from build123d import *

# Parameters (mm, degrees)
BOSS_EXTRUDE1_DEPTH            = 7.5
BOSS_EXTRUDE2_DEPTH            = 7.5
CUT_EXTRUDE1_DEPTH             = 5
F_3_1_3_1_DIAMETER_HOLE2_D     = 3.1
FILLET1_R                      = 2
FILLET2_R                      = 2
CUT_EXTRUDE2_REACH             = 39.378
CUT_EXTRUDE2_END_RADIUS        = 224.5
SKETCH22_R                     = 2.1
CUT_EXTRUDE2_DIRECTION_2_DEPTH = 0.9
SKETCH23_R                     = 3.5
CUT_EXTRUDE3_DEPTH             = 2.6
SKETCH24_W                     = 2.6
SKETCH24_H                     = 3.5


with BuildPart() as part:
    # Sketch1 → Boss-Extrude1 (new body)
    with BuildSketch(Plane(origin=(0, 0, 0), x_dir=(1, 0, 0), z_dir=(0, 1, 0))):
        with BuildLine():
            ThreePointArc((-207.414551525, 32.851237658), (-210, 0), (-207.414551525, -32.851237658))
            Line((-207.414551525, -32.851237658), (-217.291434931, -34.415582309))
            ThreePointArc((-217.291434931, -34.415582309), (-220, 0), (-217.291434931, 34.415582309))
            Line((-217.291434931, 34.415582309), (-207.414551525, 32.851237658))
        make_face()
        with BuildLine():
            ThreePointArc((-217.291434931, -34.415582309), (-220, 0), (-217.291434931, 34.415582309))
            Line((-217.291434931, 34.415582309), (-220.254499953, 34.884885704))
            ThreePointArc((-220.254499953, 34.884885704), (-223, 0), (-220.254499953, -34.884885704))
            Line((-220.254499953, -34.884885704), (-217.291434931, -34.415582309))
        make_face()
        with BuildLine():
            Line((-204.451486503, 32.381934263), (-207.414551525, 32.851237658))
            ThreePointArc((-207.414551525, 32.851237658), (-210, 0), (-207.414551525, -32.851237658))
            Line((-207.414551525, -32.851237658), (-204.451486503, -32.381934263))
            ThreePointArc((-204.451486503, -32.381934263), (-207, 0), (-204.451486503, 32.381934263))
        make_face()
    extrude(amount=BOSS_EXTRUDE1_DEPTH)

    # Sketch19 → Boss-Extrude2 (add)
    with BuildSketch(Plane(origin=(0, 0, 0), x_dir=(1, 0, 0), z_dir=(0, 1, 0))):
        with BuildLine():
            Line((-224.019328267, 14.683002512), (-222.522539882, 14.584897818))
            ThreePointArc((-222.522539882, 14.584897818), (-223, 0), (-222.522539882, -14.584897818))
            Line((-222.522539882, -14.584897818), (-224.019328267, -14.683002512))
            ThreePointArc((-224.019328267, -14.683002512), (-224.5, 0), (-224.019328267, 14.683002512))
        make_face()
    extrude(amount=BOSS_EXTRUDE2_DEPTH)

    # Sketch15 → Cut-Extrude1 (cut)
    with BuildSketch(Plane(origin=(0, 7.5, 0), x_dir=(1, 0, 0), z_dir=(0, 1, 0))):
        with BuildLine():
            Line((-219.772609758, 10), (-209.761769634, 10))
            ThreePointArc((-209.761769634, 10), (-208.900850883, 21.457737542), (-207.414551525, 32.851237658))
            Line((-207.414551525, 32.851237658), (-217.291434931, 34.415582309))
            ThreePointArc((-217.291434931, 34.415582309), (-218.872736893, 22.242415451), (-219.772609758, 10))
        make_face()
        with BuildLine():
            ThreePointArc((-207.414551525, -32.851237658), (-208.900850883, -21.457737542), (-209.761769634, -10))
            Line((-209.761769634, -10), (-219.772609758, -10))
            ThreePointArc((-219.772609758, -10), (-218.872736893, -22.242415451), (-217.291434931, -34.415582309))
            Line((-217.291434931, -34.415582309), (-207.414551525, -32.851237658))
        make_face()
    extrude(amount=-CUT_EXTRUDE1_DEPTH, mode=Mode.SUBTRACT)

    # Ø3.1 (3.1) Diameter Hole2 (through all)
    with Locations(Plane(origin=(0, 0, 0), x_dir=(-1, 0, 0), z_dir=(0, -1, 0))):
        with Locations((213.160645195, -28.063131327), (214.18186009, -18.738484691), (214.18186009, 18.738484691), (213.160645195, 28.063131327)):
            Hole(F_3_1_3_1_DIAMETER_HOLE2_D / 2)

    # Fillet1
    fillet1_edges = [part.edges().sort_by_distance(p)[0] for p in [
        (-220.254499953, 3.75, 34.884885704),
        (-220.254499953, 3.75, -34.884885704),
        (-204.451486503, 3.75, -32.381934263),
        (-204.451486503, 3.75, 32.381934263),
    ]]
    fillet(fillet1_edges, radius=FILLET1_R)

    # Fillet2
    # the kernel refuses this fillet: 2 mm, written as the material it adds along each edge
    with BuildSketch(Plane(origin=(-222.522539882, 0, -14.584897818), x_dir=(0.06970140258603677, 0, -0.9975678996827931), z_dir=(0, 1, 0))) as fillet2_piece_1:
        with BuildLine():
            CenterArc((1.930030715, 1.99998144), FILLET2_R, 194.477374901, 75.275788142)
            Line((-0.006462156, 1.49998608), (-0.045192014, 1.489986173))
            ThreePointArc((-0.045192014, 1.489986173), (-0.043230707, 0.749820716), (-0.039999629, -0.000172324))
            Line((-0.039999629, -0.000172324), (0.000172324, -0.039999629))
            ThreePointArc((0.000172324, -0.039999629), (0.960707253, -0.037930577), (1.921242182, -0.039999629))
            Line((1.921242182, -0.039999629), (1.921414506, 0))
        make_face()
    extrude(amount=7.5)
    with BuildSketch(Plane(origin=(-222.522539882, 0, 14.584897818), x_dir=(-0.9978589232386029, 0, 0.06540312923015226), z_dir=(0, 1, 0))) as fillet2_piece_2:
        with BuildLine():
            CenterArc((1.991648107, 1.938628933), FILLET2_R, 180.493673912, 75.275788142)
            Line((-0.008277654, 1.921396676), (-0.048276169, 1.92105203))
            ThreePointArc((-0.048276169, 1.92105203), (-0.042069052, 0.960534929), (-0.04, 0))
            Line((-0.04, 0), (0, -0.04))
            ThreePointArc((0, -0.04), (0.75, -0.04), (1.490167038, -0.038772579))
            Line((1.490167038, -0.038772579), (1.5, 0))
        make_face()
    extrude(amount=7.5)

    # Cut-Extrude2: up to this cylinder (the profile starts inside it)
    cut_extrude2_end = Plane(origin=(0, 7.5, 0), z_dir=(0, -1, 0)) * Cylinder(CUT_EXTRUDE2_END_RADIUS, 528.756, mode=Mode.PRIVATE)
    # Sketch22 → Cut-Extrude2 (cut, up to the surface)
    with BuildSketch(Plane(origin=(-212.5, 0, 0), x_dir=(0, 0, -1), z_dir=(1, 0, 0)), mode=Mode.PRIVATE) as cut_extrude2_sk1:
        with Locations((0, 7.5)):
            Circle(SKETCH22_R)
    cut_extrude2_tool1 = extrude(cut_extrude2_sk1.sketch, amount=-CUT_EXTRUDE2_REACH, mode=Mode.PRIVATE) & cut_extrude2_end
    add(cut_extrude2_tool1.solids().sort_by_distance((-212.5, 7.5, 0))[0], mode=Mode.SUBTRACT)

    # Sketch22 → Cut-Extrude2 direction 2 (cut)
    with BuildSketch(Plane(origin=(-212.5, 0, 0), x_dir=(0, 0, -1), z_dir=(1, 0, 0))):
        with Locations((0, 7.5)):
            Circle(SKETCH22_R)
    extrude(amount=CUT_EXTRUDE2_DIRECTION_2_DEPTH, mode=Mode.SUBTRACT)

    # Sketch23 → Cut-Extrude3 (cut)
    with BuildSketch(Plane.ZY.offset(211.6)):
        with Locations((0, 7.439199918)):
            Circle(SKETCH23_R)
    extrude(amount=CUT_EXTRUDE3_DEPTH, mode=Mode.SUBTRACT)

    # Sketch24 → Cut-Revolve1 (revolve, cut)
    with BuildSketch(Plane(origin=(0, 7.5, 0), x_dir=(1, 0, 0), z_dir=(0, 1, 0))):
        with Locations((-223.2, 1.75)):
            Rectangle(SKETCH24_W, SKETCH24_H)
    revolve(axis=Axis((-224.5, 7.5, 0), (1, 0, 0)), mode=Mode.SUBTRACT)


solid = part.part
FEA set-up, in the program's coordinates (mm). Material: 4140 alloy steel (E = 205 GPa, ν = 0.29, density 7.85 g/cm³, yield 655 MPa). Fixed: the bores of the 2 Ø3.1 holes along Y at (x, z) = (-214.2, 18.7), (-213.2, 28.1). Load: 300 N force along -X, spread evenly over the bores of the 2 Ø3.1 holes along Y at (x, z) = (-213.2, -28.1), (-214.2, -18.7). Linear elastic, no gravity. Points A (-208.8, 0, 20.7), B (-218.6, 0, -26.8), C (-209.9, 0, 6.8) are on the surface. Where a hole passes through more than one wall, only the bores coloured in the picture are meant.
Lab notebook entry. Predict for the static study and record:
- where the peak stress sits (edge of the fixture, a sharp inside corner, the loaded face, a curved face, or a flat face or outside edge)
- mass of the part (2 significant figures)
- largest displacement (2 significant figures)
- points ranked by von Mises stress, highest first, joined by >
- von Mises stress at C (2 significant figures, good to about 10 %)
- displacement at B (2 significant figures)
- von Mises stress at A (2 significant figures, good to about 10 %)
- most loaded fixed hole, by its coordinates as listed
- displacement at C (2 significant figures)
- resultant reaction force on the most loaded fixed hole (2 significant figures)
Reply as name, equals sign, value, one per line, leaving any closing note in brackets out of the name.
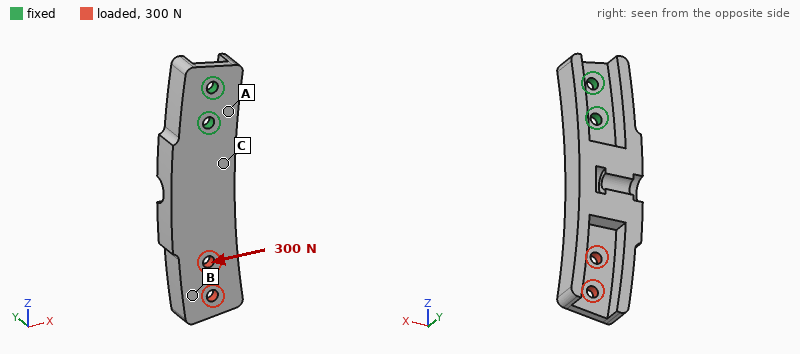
where the peak stress sits = edge of the fixture
mass of the part = 46 g
largest displacement = 52 µm
points ranked by von Mises stress, highest first, joined by > = A > C > B
von Mises stress at C = 24 MPa
displacement at B = 44 µm
von Mises stress at A = 40 MPa
most loaded fixed hole, by its coordinates as listed = (-214.2, 18.7)
displacement at C = 9.7 µm
resultant reaction force on the most loaded fixed hole = 1.2 kN
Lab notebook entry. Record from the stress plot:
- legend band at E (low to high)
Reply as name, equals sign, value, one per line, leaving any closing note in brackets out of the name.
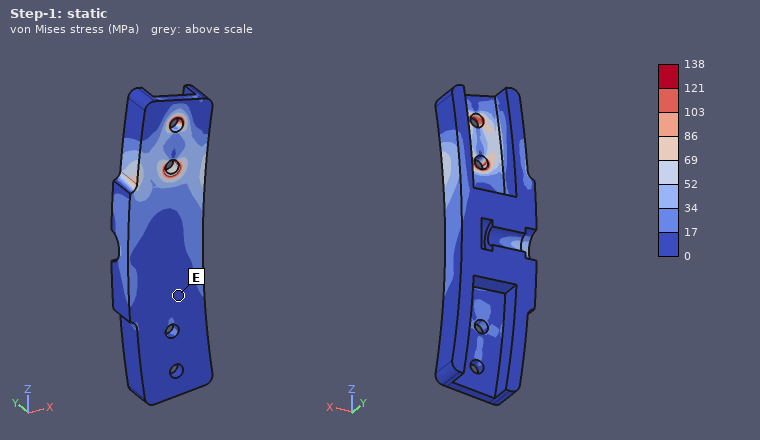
legend band at E = 0 to 17 MPa
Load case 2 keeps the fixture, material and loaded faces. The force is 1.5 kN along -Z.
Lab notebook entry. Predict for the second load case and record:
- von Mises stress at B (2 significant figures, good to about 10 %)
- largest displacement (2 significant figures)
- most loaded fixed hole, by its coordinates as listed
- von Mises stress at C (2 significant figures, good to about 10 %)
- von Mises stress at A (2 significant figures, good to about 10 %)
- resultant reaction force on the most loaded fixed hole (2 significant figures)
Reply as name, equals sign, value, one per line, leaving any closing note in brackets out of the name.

von Mises stress at B = 19 MPa
largest displacement = 44 µm
most loaded fixed hole, by its coordinates as listed = (-214.2, 18.7)
von Mises stress at C = 45 MPa
von Mises stress at A = 22 MPa
resultant reaction force on the most loaded fixed hole = 1.1 kN
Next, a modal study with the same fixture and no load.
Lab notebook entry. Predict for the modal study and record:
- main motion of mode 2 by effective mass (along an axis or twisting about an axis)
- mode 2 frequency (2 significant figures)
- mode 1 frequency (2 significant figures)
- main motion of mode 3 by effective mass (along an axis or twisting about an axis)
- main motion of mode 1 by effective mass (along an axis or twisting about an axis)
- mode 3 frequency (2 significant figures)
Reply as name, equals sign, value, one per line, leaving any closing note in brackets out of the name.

main motion of mode 2 by effective mass = along X
mode 2 frequency = 3500 Hz
mode 1 frequency = 1700 Hz
main motion of mode 3 by effective mass = twisting about Z
main motion of mode 1 by effective mass = along Y
mode 3 frequency = 5400 Hz
